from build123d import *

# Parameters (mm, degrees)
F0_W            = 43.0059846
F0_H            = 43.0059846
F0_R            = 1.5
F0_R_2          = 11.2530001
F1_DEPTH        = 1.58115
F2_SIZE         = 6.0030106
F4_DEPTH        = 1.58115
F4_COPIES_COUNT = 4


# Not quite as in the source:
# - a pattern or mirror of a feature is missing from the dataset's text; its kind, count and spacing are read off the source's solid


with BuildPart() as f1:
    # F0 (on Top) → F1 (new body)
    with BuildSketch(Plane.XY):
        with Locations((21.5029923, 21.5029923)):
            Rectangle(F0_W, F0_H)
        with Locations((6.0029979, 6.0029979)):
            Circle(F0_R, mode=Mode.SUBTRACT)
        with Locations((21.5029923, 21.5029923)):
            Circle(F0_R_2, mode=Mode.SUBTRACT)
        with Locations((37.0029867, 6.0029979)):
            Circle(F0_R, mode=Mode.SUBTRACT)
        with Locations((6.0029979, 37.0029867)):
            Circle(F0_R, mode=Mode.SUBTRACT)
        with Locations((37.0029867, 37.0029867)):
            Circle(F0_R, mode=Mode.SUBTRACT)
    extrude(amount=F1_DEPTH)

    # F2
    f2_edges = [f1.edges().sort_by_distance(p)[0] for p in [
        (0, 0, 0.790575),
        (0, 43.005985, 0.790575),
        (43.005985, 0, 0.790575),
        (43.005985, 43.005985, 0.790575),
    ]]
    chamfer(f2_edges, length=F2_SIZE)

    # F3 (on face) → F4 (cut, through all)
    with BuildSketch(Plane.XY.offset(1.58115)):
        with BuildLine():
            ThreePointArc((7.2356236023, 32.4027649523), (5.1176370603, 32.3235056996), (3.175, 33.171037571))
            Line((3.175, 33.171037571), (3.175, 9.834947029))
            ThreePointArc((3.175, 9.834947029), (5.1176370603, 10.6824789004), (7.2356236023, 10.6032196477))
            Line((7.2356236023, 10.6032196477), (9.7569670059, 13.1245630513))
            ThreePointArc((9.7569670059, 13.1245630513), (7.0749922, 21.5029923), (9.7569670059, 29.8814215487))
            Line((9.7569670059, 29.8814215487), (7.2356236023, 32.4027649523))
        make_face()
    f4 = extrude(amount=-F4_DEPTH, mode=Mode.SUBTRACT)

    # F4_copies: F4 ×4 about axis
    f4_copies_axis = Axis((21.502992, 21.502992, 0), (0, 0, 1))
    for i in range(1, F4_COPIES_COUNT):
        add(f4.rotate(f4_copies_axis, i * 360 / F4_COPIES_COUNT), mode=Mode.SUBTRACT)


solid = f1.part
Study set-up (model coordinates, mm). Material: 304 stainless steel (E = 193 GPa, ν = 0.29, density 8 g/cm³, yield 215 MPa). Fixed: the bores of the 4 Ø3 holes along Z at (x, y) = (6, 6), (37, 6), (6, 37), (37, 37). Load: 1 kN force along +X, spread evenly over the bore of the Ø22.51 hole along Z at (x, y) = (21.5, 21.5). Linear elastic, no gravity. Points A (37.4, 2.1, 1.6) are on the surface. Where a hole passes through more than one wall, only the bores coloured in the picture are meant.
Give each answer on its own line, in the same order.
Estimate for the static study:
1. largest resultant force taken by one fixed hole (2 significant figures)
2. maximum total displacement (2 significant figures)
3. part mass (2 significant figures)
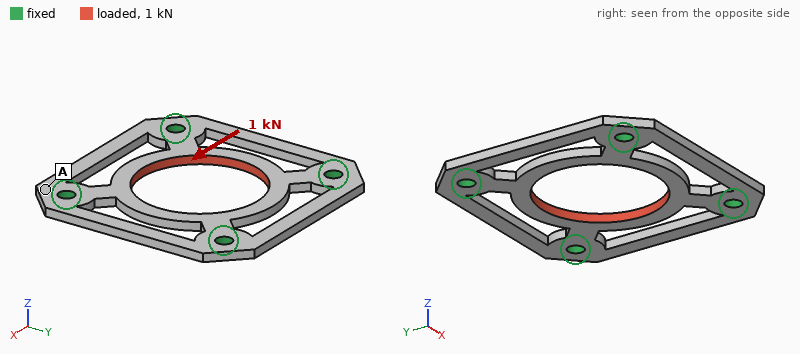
250 N
15 µm
12 g
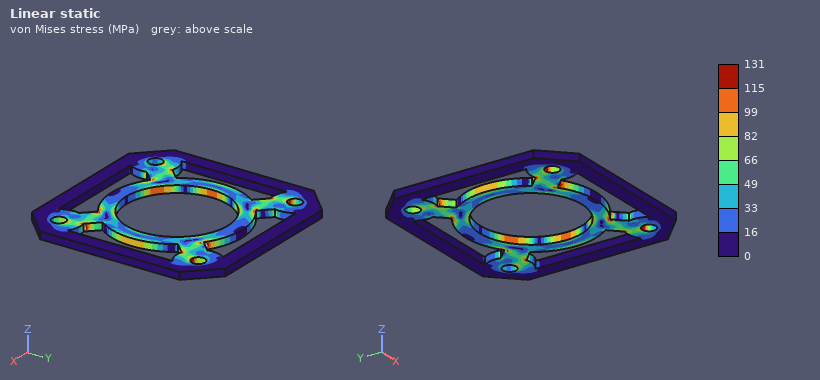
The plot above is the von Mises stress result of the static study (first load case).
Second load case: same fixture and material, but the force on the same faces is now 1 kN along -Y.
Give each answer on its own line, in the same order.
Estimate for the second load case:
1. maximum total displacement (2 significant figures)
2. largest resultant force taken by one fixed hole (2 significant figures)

15 µm
250 N
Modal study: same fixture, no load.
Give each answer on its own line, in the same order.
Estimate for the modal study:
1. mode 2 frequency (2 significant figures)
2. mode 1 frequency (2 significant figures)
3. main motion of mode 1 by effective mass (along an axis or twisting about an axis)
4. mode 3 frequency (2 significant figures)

9000 Hz
8300 Hz
along Z
9000 Hz
